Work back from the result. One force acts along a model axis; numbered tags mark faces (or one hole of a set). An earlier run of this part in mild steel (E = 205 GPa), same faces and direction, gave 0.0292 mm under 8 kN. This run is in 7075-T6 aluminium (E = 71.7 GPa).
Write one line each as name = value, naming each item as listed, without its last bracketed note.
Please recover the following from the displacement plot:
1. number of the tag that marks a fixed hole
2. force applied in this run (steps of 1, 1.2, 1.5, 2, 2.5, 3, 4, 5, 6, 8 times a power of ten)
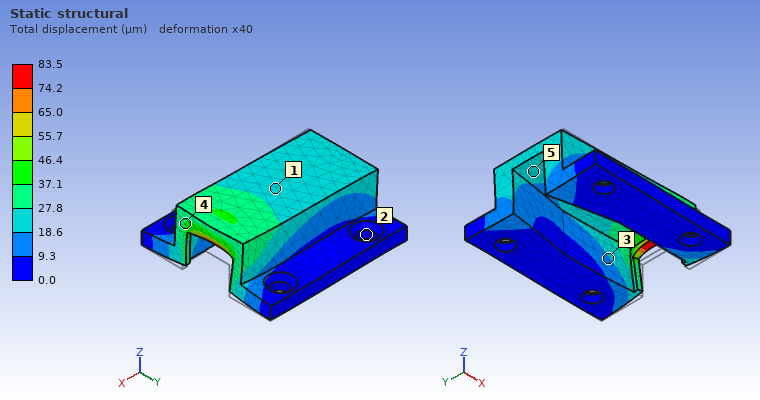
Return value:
number of the tag that marks a fixed hole = 2
force applied in this run = 8 kN
